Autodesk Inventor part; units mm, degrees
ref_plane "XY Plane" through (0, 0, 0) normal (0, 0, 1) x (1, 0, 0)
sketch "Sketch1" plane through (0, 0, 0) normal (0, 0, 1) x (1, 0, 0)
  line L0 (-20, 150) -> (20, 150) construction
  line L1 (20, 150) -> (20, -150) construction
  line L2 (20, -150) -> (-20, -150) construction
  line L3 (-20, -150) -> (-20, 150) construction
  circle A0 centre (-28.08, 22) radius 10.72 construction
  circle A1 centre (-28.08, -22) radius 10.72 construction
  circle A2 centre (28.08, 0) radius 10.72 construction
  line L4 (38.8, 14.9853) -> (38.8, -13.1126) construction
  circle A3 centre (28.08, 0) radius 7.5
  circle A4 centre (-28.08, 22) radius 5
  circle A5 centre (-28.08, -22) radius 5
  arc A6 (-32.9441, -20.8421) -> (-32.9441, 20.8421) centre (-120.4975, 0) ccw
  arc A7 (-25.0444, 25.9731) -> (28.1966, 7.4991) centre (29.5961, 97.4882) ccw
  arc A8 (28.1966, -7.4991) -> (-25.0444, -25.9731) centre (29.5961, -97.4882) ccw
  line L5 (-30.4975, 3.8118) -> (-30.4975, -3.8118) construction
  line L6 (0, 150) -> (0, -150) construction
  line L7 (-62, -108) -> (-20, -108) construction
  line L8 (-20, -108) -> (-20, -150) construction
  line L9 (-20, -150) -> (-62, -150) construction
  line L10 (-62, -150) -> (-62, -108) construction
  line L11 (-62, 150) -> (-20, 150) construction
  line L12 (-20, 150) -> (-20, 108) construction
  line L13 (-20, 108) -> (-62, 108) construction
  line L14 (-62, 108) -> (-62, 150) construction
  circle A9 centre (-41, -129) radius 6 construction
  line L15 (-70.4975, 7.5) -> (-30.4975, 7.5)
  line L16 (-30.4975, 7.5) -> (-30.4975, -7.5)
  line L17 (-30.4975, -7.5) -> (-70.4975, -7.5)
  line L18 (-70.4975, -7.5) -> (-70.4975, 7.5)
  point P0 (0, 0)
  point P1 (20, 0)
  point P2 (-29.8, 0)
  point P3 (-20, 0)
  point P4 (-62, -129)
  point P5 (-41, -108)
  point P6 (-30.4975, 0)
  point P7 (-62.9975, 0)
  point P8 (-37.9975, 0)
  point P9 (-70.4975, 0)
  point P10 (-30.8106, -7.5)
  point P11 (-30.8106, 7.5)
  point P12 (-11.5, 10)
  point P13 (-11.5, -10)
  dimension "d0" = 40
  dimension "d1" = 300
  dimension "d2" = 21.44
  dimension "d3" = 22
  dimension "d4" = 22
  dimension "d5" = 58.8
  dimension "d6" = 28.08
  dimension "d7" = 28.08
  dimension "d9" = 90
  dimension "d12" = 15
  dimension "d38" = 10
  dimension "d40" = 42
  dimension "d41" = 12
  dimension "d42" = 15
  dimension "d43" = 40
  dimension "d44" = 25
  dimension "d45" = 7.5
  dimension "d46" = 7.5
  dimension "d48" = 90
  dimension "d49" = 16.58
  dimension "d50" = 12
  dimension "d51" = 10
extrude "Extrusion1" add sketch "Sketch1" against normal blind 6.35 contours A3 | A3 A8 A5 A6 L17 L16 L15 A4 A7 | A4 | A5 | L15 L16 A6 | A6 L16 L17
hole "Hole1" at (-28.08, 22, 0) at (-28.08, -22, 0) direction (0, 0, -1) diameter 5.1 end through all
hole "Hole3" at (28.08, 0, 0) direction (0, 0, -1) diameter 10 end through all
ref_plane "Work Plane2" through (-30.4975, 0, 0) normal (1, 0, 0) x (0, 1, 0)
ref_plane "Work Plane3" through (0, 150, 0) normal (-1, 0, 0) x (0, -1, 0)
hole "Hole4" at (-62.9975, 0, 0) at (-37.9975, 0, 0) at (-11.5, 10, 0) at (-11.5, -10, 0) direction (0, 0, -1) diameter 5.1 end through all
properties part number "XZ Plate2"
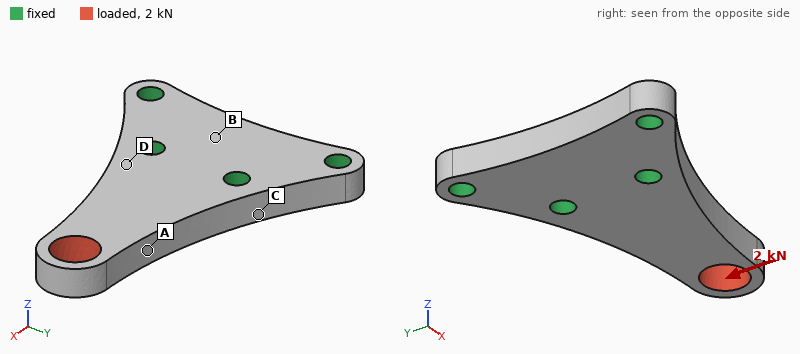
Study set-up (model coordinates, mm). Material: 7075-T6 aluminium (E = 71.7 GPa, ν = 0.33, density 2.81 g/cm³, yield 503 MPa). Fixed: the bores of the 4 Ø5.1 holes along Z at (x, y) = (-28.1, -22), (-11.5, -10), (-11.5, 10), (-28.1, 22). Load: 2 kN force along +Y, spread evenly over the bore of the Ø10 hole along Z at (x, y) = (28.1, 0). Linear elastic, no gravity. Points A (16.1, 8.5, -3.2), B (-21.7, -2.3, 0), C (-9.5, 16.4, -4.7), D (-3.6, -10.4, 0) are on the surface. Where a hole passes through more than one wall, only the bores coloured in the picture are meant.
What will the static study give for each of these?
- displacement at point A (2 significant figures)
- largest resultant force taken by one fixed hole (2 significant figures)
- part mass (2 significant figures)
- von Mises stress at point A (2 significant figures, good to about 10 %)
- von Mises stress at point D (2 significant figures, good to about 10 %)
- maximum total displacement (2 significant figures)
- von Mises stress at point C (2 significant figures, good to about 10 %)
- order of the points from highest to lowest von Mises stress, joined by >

0.051 mm
3.4 kN
31 g
93 MPa
67 MPa
0.17 mm
36 MPa
A > D > C > B
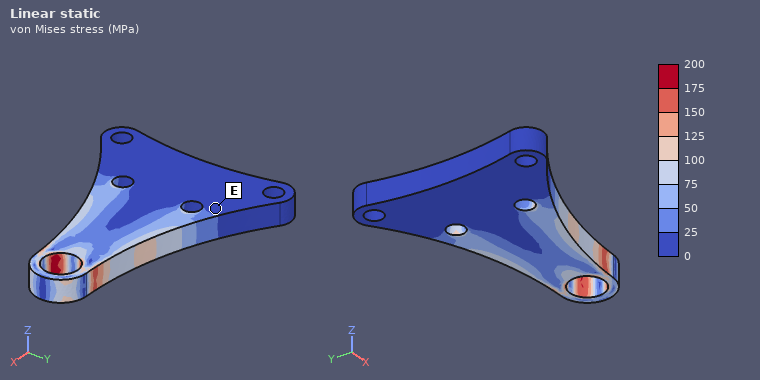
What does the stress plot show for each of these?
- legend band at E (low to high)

0 to 25 MPa
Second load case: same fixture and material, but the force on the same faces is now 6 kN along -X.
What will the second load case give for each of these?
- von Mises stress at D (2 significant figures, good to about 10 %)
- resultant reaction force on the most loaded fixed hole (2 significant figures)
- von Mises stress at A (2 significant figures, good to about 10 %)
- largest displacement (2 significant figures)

39 MPa
2.9 kN
80 MPa
63 µm
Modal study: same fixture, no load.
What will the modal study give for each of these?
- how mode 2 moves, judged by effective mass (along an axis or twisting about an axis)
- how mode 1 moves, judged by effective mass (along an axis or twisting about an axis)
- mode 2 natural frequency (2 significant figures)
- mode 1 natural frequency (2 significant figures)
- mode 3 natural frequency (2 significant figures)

along Y
along Z
12 kHz
3800 Hz
16 kHz
